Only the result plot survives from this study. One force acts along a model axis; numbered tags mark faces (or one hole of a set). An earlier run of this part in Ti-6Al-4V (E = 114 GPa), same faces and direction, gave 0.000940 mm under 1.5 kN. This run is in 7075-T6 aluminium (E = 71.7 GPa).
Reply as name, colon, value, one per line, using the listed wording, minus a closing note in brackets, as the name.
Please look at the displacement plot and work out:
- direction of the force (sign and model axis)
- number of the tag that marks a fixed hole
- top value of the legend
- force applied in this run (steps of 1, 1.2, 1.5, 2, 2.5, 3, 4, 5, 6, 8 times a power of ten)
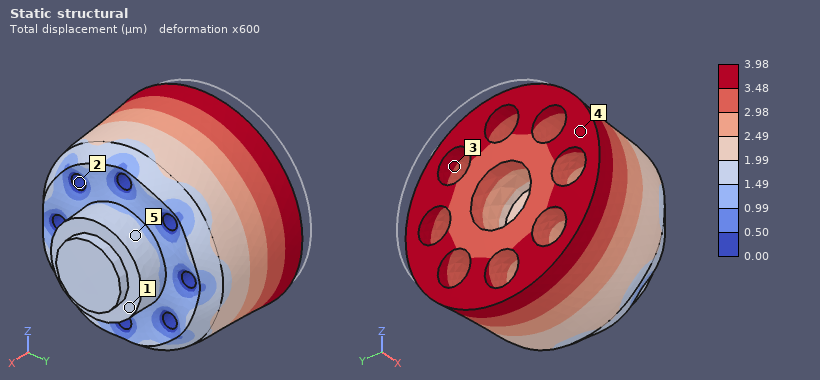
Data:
direction of the force: +X
number of the tag that marks a fixed hole: 2
top value of the legend: 3.98 µm
force applied in this run: 4 kN
